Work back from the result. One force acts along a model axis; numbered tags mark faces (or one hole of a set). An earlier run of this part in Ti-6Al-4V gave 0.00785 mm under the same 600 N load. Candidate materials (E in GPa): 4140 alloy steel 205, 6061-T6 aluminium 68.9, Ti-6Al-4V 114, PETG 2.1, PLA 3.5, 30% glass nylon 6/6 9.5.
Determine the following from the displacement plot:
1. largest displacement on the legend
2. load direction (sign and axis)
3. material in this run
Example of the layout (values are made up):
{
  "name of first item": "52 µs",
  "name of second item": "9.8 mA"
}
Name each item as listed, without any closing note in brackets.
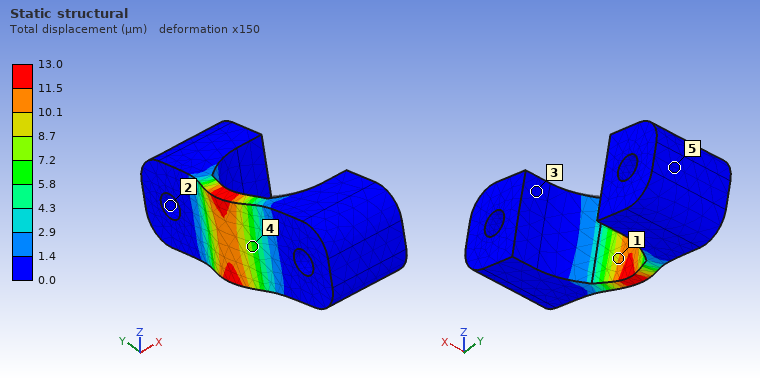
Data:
{
  "largest displacement on the legend": "13.0 µm",
  "load direction": "-X",
  "material in this run": "6061-T6 aluminium"
}
